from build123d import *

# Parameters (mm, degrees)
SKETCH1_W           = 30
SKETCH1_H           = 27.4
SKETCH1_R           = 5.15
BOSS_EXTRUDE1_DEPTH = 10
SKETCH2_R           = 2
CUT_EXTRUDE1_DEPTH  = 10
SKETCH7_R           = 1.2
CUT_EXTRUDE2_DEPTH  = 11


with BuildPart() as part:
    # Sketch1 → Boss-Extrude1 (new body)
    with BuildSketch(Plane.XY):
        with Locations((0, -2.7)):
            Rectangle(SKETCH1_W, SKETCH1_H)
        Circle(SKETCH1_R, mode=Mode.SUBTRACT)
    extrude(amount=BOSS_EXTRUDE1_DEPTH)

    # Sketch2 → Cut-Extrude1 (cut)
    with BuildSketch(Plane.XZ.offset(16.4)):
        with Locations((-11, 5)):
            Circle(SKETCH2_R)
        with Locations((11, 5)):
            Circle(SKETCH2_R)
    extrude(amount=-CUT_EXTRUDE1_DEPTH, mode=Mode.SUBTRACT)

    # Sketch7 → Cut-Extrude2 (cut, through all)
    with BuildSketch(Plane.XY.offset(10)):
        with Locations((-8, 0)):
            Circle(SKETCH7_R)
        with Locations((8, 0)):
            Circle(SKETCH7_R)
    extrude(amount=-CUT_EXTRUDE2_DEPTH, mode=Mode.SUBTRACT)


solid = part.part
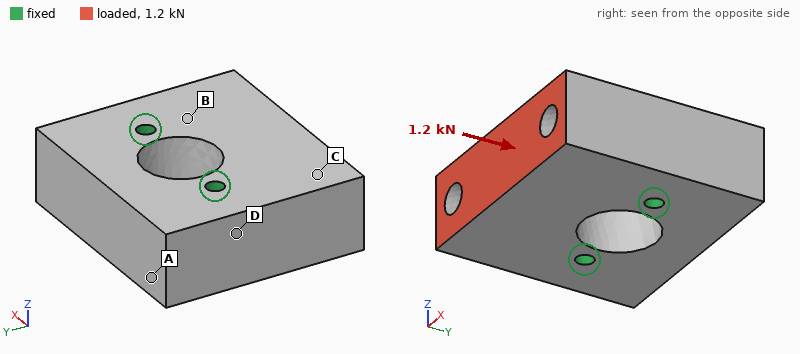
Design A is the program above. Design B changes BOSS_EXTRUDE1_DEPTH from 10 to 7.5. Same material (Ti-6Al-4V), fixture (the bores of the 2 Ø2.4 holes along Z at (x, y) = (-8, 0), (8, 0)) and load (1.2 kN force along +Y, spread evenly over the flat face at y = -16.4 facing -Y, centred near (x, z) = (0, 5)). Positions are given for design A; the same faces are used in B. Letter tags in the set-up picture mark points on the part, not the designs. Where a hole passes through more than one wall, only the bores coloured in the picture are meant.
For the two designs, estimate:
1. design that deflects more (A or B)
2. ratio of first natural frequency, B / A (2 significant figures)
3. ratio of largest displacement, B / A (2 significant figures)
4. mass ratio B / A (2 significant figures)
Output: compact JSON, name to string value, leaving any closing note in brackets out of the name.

{"design that deflects more": "B", "ratio of first natural frequency, B / A": "0.83", "ratio of largest displacement, B / A": "1.4", "mass ratio B / A": "0.74"}
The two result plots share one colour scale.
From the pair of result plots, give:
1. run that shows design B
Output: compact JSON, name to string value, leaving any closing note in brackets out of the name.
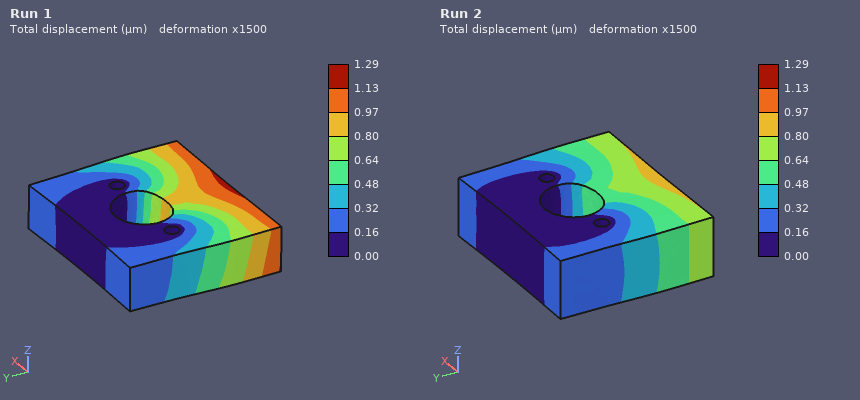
{"run that shows design B": "Run 1"}
